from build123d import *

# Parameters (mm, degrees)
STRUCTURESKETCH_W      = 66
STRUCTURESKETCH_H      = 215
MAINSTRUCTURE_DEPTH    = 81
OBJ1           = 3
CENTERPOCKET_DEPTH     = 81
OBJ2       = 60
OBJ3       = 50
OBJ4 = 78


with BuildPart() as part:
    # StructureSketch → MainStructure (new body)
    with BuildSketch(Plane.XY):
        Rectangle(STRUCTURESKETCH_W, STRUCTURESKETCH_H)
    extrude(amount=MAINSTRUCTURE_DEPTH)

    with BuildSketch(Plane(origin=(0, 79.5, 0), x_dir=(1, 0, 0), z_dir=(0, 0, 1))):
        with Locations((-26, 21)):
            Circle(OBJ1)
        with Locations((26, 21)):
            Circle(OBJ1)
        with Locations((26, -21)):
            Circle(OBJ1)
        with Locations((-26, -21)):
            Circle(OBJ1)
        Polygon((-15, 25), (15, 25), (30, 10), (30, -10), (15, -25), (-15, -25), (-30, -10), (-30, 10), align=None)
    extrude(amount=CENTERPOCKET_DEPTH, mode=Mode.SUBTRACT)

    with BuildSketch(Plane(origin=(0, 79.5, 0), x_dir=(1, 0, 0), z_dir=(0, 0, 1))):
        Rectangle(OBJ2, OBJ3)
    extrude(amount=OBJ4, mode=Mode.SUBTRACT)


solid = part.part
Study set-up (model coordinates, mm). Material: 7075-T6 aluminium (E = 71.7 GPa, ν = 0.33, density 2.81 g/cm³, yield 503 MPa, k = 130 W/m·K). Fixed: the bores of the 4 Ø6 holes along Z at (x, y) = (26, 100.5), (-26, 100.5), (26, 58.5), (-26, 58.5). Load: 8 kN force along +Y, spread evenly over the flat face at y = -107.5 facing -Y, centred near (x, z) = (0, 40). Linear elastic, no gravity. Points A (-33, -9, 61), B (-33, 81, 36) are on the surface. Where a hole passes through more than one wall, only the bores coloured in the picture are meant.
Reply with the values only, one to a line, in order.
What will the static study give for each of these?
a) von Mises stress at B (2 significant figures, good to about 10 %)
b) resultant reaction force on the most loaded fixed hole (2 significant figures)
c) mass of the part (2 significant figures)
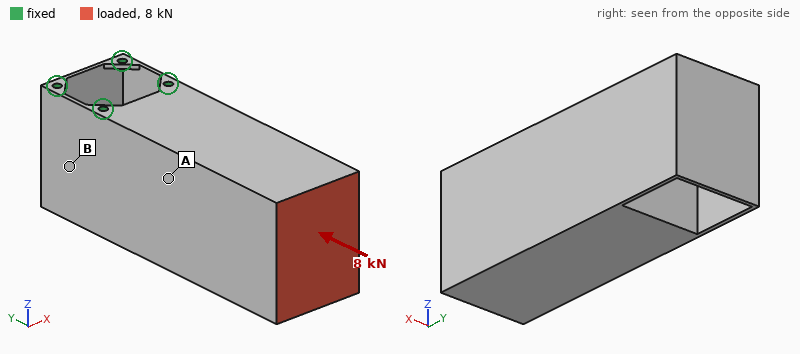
26 MPa
4.2 kN
2.5 kg
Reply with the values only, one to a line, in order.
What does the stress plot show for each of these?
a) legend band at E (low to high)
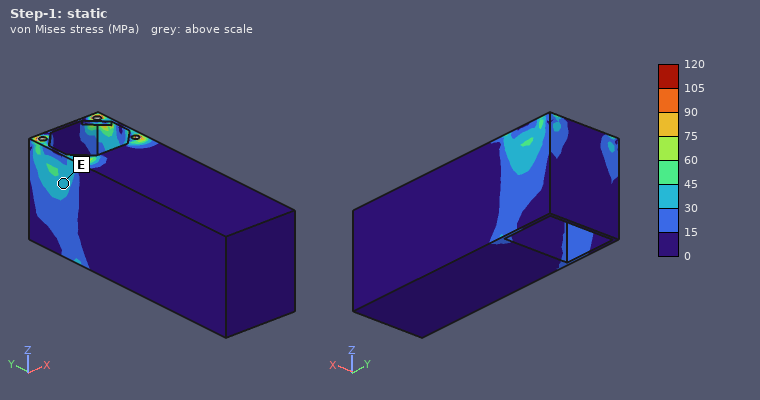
30 to 45 MPa
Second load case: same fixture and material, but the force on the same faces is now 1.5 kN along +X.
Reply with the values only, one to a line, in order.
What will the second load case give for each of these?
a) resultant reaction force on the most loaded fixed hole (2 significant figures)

3.9 kN
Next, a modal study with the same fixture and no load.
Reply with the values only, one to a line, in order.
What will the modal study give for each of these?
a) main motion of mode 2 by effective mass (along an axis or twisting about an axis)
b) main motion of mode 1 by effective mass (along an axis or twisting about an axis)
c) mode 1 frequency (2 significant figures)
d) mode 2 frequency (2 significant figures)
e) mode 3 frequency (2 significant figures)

along X
along Z
390 Hz
710 Hz
1400 Hz
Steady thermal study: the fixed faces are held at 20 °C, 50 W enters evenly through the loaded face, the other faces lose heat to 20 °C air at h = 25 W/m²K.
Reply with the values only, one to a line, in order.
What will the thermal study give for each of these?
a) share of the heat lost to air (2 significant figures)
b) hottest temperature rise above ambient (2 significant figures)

46 %
20 K
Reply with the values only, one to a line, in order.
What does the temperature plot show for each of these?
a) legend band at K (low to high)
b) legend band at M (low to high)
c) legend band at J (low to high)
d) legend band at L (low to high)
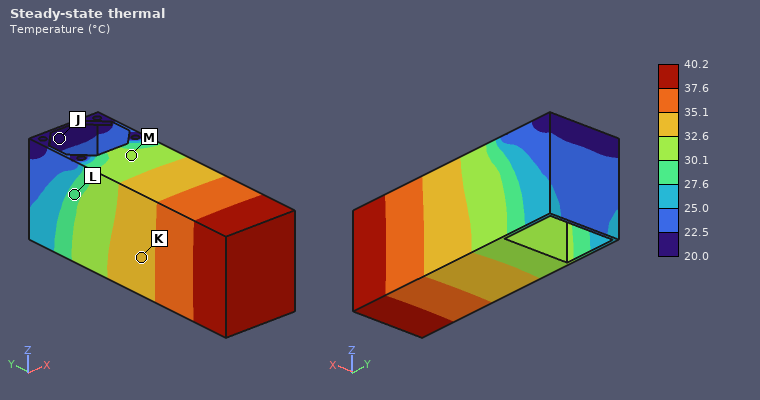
32.6 to 35.1 °C
30.1 to 32.6 °C
20.0 to 22.5 °C
27.6 to 30.1 °C
